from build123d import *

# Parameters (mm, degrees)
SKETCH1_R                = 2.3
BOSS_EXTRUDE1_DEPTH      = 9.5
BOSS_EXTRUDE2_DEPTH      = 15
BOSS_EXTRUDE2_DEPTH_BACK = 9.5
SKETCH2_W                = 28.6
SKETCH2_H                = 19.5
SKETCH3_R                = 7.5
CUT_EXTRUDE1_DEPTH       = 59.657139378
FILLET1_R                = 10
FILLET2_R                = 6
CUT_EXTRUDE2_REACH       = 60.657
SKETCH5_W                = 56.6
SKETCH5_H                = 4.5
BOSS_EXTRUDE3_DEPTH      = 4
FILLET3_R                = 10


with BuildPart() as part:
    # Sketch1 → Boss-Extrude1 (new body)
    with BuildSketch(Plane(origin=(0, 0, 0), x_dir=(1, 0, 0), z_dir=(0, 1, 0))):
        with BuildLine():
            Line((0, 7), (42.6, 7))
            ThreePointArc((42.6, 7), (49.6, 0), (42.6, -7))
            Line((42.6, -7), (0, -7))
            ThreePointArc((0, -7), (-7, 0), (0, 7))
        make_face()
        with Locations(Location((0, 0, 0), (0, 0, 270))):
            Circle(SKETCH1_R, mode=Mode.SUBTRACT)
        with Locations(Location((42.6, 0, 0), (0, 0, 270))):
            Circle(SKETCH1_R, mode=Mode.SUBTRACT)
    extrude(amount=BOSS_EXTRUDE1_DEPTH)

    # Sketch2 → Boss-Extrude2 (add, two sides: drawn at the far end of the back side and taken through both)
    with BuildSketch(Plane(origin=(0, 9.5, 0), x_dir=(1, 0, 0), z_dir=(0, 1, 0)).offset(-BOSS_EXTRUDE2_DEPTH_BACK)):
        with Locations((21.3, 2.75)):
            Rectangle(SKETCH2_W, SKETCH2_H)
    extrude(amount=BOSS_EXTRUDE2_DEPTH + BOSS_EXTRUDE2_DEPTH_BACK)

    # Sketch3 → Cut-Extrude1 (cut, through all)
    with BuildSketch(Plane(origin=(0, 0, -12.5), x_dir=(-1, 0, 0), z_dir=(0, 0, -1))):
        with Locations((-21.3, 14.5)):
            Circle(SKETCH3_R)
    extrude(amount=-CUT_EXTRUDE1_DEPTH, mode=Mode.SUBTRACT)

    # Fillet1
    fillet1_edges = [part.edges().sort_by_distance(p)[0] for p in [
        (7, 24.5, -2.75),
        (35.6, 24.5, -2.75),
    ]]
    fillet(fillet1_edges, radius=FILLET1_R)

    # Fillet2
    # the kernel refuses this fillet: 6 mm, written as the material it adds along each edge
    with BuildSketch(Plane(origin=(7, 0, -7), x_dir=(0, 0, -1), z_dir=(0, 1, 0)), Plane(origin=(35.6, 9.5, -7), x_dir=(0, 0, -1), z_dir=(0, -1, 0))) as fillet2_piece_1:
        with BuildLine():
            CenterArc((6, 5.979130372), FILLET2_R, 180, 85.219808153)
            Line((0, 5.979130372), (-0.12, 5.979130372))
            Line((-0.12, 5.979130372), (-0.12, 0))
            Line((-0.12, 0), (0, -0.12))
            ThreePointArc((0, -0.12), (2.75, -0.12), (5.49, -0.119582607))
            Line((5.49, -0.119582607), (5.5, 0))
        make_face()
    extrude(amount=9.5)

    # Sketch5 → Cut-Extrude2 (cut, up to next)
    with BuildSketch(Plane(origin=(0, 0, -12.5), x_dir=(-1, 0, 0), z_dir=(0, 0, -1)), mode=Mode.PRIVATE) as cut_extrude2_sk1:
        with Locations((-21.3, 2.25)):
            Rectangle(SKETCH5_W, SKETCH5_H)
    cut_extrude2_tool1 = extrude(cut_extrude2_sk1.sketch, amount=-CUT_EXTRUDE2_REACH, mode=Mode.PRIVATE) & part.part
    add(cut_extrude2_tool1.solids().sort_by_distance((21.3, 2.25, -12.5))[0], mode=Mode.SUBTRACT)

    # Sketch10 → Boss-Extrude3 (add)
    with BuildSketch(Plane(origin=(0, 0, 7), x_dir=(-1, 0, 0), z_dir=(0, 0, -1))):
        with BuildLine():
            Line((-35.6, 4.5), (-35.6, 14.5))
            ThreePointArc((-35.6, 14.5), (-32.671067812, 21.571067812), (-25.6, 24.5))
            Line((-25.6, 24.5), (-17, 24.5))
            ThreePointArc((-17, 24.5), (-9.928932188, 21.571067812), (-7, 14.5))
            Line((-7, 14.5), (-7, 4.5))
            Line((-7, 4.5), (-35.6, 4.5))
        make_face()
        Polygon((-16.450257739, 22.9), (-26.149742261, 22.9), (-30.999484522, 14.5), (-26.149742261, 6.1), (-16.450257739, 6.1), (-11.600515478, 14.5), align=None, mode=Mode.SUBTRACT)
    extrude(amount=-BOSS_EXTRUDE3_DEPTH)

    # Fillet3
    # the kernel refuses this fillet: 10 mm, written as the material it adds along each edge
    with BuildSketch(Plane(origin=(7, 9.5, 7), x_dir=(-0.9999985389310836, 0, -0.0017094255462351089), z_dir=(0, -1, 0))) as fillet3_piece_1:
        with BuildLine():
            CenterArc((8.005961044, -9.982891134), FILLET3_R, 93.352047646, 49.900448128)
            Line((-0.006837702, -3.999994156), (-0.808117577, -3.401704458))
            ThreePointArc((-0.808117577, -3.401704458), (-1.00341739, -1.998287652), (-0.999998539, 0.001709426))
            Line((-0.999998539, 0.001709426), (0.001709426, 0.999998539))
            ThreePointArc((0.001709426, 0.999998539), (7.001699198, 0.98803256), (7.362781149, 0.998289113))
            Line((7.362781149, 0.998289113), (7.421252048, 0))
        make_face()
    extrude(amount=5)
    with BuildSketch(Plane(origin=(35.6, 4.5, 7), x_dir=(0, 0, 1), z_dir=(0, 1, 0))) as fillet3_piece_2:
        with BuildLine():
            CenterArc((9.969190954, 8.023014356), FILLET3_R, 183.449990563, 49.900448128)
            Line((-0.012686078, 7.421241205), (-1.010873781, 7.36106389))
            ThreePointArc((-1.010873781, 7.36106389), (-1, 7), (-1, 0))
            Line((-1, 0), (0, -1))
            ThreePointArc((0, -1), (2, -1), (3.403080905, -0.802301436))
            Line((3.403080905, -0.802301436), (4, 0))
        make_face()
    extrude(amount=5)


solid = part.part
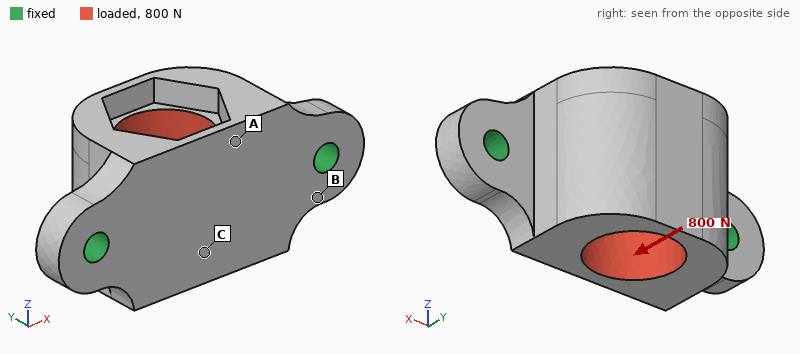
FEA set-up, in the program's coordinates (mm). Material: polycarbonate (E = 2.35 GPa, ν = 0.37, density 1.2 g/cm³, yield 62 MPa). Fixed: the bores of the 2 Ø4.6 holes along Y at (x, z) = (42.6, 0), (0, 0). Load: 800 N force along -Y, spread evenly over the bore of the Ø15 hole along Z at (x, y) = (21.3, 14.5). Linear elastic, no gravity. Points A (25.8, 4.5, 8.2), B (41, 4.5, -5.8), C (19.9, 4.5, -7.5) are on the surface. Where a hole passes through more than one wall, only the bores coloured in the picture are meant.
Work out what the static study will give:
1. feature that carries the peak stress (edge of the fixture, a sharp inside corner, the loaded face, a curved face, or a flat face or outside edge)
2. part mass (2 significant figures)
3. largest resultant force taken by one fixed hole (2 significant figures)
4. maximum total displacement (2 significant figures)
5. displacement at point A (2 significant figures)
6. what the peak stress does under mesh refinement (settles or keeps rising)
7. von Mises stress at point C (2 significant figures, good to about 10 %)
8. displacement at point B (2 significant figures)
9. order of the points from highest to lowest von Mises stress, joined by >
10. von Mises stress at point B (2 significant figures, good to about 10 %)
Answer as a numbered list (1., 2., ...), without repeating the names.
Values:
1. edge of the fixture
2. 12 g
3. 410 N
4. 0.39 mm
5. 0.069 mm
6. keeps rising
7. 8.6 MPa
8. 0.074 mm
9. B > C > A
10. 17 MPa
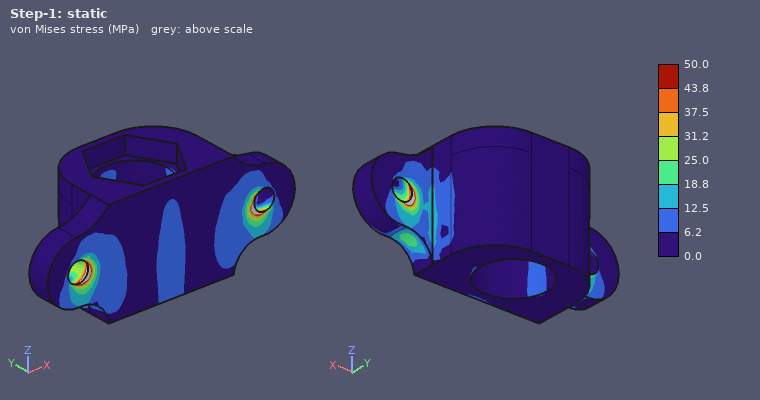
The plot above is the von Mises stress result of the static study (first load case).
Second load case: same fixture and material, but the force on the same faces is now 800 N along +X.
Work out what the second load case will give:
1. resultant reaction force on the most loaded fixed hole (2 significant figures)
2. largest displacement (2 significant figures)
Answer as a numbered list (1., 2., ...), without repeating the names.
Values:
1. 430 N
2. 0.14 mm
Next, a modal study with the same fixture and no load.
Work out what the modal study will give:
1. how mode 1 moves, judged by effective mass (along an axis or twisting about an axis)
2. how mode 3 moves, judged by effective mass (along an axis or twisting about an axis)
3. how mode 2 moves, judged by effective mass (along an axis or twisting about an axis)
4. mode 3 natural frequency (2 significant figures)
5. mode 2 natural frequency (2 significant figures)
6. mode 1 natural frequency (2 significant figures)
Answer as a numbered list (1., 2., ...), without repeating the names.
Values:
1. along Z
2. along X
3. along Y
4. 4700 Hz
5. 3800 Hz
6. 1800 Hz
